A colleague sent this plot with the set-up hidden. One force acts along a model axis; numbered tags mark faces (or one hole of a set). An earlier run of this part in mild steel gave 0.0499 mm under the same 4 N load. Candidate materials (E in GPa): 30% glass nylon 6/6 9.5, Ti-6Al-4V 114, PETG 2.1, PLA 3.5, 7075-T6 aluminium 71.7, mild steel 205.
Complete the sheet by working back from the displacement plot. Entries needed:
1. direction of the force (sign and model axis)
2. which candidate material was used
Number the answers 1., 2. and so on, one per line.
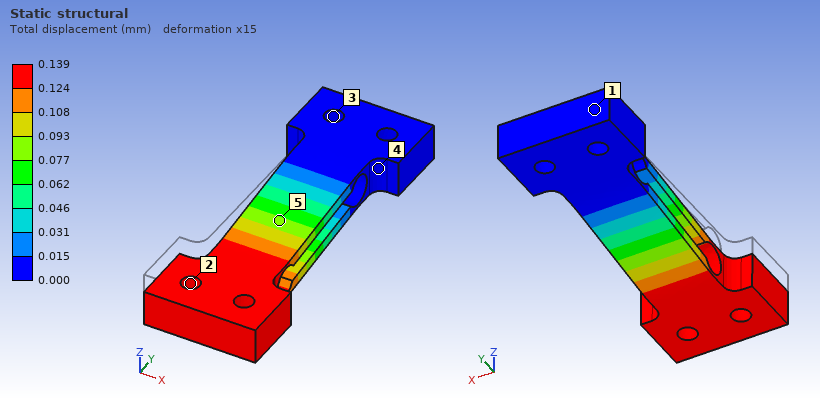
1. -Z
2. 7075-T6 aluminium
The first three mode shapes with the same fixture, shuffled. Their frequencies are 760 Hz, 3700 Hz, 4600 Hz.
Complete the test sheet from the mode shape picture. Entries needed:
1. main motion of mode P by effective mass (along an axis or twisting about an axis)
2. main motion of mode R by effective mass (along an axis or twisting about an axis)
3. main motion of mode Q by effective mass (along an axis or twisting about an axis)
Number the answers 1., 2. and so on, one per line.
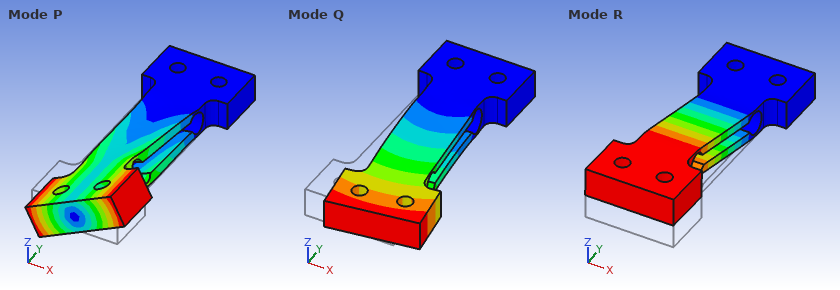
1. twisting about Y
2. along Z
3. along X
